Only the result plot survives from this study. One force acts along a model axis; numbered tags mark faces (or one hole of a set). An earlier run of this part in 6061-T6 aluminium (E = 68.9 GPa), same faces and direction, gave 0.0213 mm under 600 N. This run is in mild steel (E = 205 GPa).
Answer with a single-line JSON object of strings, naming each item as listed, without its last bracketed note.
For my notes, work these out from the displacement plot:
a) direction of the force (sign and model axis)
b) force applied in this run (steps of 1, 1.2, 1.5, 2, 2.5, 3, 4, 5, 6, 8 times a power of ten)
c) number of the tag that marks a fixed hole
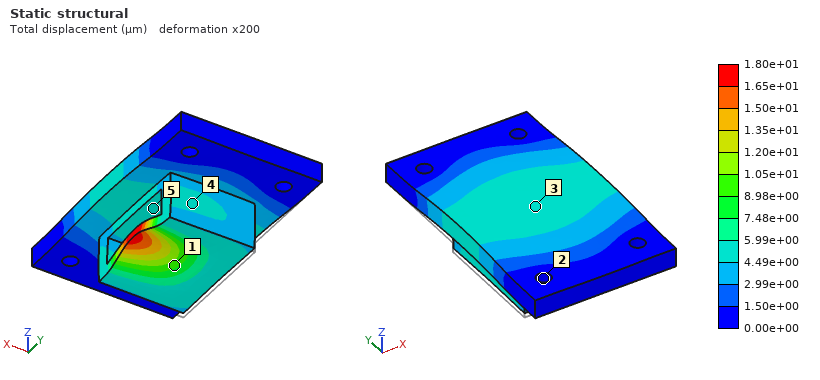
{"direction of the force": "+Z", "force applied in this run": "1.5 kN", "number of the tag that marks a fixed hole": "2"}
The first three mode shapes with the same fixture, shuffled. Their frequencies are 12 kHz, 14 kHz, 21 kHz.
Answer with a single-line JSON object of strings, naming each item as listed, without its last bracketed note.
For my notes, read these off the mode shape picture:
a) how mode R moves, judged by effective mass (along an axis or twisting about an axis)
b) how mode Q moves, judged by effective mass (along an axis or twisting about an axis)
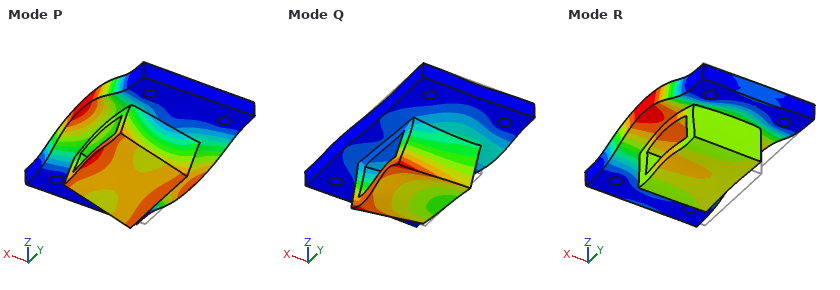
{"how mode R moves, judged by effective mass": "along Z", "how mode Q moves, judged by effective mass": "along Y"}
